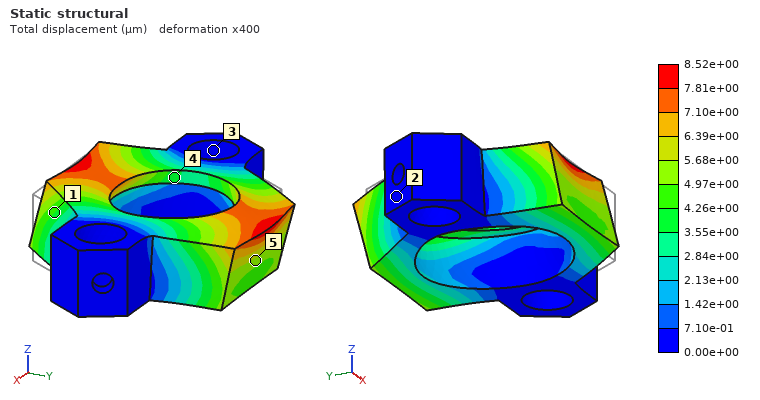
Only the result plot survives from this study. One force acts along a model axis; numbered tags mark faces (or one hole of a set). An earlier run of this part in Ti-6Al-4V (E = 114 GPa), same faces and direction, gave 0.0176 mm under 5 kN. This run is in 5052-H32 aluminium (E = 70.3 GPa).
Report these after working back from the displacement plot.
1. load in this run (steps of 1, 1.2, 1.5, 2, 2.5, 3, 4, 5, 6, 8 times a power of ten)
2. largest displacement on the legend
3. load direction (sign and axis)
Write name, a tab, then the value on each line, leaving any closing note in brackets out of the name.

load in this run	1.5 kN
largest displacement on the legend	8.52e+00 µm
load direction	+Y
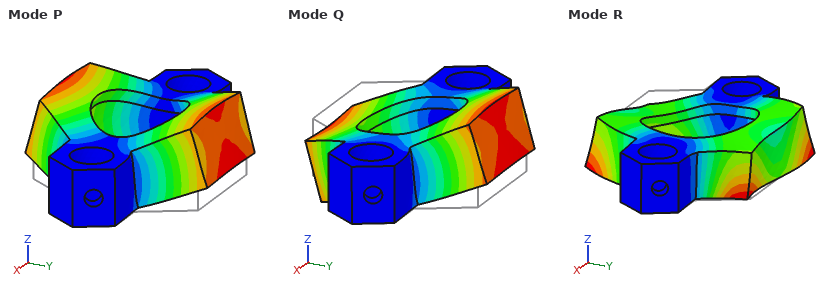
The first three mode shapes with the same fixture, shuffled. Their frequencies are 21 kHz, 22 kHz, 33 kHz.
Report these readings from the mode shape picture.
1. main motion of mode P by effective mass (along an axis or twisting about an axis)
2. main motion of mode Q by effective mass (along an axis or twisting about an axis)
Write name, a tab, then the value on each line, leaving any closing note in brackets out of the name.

main motion of mode P by effective mass	along Z
main motion of mode Q by effective mass	twisting about X
